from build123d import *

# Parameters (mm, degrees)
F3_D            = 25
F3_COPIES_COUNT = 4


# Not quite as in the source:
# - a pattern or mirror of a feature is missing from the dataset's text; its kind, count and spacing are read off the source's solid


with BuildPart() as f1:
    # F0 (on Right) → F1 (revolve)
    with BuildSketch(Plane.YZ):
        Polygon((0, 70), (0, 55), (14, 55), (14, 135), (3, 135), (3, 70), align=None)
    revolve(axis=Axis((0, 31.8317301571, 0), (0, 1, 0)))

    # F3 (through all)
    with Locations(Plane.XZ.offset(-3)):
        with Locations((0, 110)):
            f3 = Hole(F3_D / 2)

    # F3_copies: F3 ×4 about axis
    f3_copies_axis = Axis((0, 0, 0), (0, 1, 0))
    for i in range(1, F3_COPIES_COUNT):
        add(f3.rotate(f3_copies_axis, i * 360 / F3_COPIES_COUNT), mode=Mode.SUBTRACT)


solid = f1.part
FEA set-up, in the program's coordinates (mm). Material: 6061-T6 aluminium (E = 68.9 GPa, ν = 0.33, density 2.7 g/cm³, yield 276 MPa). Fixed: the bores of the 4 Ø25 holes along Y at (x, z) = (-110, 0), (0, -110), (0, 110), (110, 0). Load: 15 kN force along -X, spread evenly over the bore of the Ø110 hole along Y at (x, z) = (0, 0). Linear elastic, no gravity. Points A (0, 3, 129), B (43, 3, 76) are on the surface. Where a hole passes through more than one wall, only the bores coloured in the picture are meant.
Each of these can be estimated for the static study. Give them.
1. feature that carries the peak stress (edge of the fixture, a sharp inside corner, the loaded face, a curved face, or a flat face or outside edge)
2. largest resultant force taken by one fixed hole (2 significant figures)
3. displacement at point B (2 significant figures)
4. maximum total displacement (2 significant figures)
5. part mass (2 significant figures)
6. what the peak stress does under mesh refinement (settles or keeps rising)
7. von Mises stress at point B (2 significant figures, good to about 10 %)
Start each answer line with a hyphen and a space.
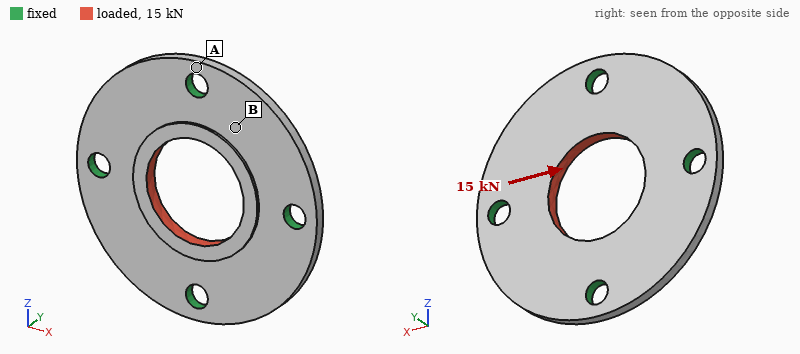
- edge of the fixture
- 4.3 kN
- 4.4 µm
- 7.4 µm
- 1.4 kg
- keeps rising
- 2.7 MPa
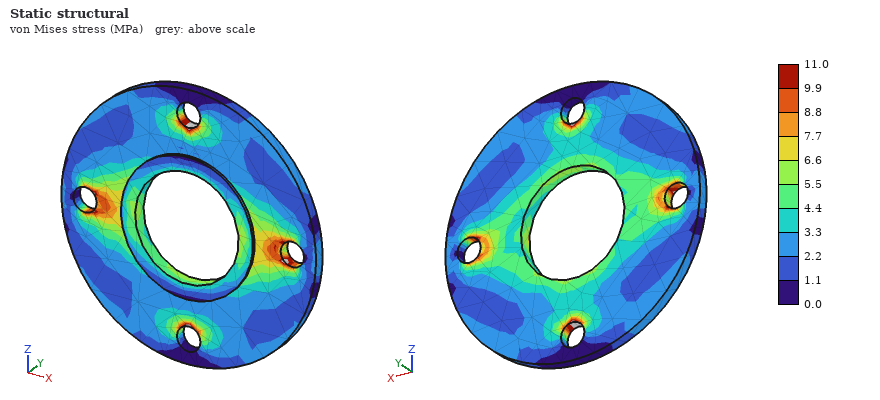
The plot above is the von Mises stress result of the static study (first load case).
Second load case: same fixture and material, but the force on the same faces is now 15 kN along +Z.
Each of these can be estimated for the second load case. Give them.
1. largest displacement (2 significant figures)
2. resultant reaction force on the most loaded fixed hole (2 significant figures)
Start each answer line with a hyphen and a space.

- 7.4 µm
- 4.3 kN
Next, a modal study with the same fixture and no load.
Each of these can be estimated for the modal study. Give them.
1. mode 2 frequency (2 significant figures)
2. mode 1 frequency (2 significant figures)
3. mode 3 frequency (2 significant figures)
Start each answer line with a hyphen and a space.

- 2200 Hz
- 2200 Hz
- 2200 Hz
